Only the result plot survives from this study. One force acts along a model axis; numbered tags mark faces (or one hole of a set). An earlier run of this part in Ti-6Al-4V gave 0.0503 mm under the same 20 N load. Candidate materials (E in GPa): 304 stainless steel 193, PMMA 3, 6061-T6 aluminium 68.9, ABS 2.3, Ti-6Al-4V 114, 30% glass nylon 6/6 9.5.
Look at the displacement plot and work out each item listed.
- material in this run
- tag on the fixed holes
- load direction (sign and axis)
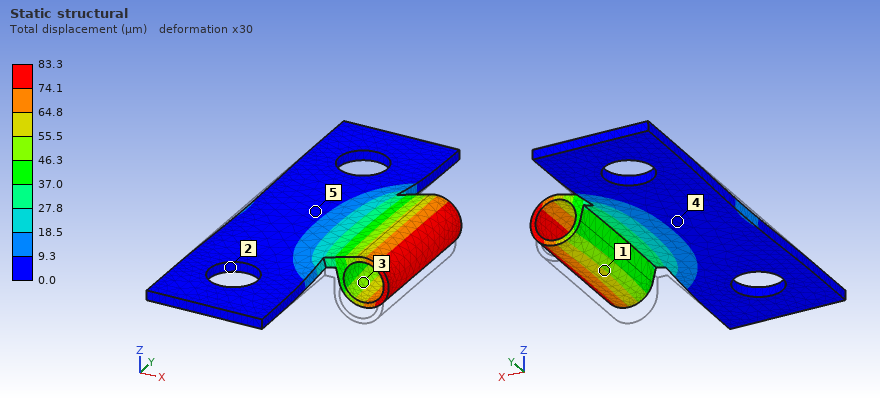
6061-T6 aluminium
2
+Z
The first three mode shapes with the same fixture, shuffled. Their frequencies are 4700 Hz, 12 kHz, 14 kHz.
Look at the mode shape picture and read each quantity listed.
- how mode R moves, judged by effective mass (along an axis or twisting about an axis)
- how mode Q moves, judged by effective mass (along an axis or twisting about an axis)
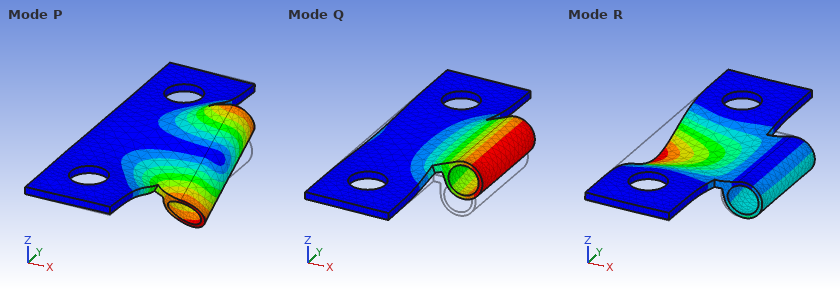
along Z
along Z
